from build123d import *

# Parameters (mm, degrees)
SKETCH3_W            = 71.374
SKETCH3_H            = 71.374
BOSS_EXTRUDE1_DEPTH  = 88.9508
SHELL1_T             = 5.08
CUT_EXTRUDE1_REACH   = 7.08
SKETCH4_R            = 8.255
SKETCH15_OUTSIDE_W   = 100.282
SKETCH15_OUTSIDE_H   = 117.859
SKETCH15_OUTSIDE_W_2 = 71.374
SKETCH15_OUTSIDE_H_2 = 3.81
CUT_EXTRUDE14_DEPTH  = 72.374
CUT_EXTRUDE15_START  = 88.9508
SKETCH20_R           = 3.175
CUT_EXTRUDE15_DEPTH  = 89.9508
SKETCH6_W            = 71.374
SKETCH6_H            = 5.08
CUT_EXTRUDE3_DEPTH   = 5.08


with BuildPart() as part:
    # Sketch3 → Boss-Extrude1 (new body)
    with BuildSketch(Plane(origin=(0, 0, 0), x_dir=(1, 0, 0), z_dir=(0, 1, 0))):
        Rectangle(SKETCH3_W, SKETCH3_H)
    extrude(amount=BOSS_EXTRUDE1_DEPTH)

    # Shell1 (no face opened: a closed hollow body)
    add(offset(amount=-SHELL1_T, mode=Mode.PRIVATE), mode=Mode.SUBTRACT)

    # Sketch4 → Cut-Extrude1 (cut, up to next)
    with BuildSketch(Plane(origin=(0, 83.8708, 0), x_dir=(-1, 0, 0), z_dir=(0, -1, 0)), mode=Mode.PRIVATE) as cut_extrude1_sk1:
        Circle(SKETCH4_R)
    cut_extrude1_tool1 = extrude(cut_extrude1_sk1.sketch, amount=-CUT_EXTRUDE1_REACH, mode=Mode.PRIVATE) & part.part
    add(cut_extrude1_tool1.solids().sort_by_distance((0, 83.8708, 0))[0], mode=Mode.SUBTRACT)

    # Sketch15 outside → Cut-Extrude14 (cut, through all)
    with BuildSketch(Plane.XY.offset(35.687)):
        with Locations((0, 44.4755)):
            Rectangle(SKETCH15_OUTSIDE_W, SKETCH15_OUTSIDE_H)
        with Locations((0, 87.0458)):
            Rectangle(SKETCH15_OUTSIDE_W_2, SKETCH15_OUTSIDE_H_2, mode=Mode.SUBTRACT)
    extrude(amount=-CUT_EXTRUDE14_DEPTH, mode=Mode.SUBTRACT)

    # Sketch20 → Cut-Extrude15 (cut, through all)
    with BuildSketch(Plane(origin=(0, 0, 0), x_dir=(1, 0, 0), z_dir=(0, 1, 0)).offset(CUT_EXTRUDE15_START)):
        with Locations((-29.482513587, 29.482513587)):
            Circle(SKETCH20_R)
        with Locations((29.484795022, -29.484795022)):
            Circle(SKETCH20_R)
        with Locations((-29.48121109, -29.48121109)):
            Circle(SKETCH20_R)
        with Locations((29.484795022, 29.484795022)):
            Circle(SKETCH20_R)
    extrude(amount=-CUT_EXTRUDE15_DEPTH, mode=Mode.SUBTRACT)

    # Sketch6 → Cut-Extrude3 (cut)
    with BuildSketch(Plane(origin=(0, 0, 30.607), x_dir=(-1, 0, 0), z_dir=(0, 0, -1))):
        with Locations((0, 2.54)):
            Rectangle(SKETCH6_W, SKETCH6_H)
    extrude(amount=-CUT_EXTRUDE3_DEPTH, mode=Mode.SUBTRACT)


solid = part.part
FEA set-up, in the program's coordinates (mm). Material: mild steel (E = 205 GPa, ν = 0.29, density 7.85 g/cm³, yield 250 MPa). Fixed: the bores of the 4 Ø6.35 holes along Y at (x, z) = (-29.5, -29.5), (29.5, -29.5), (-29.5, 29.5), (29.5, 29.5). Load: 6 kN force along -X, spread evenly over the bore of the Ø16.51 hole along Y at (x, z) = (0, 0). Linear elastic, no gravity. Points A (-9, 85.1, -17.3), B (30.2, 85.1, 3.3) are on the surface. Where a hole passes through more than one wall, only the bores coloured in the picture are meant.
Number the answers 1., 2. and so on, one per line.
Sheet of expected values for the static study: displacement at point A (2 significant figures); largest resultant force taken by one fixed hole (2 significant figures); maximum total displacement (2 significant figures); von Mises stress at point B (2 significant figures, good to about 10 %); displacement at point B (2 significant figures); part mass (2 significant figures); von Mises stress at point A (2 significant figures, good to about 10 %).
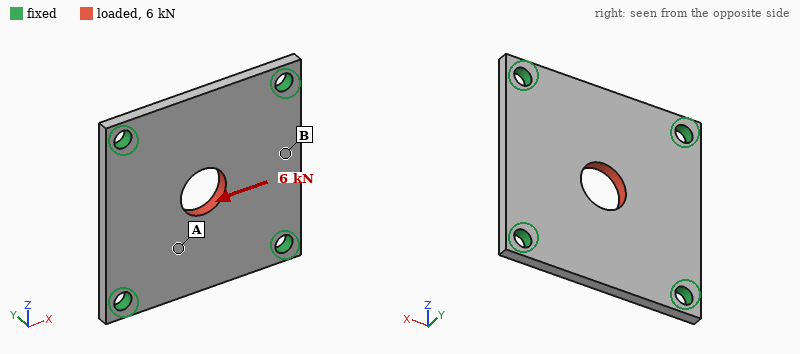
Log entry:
1. 2.8 µm
2. 1.7 kN
3. 5.5 µm
4. 8.9 MPa
5. 3.9 µm
6. 140 g
7. 21 MPa
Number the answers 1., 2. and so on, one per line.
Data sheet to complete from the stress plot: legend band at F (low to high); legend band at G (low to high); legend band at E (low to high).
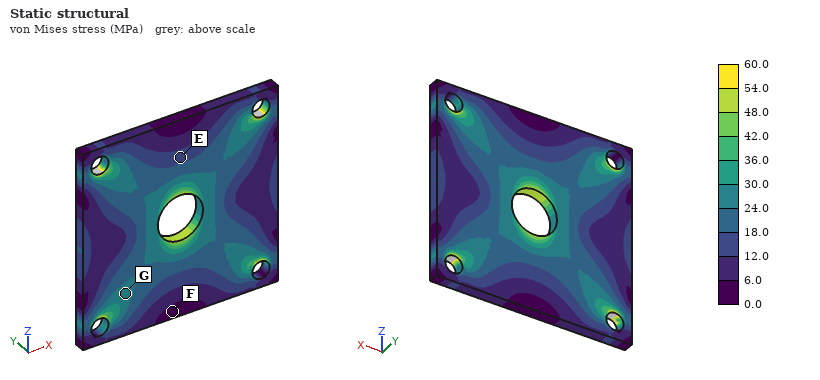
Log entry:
1. 0.0 to 6.0 MPa
2. 24.0 to 30.0 MPa
3. 12.0 to 18.0 MPa
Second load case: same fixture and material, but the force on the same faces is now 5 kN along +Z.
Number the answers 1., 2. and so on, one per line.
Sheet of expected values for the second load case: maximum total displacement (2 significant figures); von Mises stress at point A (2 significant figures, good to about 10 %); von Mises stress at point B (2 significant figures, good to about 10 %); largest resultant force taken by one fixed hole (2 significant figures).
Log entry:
1. 4.6 µm
2. 18 MPa
3. 5.4 MPa
4. 1.4 kN
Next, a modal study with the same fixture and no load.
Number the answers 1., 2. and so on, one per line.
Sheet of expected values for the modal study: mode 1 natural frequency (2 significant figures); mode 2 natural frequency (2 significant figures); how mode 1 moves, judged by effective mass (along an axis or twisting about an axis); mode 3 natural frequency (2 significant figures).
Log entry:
1. 4200 Hz
2. 6800 Hz
3. along Y
4. 6800 Hz
